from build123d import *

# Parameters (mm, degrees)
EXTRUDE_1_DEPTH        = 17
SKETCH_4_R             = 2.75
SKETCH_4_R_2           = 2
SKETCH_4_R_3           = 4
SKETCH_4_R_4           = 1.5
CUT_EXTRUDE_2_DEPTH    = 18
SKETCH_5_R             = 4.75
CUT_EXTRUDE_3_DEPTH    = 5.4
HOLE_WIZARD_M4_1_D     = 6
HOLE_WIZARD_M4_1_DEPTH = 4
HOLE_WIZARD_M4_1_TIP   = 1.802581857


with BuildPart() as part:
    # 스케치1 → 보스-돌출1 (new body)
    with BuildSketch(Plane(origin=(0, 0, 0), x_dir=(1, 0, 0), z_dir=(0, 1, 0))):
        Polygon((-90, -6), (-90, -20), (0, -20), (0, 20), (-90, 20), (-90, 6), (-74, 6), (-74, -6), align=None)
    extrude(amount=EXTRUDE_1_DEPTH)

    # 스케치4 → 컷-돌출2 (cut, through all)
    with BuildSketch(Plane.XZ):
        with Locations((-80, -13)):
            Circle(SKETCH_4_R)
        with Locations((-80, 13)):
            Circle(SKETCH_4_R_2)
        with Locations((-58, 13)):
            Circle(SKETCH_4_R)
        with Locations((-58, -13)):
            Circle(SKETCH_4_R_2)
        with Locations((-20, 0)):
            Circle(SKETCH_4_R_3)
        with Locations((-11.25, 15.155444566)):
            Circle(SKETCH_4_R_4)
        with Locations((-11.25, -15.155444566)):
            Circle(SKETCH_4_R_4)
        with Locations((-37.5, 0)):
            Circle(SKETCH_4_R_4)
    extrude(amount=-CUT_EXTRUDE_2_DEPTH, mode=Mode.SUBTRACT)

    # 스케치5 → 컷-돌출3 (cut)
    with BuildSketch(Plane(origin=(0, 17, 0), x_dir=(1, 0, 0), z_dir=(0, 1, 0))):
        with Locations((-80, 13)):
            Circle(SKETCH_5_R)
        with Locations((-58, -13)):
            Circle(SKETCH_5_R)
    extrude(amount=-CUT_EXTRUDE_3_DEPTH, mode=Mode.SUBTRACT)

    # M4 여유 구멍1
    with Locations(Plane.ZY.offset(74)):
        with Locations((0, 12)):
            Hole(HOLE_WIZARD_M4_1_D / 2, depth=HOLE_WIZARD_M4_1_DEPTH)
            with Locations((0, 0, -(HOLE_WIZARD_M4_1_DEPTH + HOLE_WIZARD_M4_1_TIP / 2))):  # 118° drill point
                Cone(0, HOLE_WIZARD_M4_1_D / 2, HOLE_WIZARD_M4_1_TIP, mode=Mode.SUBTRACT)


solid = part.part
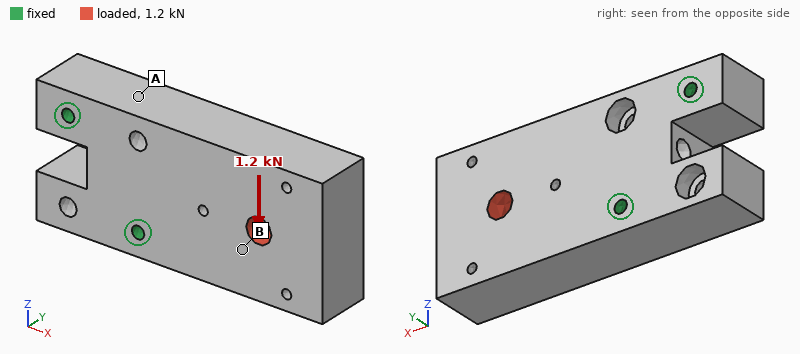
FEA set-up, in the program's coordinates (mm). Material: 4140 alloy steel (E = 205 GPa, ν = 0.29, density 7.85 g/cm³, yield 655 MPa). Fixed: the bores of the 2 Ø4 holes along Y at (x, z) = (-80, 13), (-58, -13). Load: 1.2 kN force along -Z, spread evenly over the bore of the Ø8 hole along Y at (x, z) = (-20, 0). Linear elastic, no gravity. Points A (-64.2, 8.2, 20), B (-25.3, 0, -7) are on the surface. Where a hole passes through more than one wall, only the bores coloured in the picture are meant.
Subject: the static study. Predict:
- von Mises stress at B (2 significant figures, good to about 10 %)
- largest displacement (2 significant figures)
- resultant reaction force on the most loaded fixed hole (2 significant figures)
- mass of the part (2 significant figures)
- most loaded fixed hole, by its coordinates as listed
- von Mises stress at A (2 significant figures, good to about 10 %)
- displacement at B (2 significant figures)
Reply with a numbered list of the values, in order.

1. 3.6 MPa
2. 6.0 µm
3. 2.0 kN
4. 430 g
5. (-58, -13)
6. 13 MPa
7. 3.2 µm
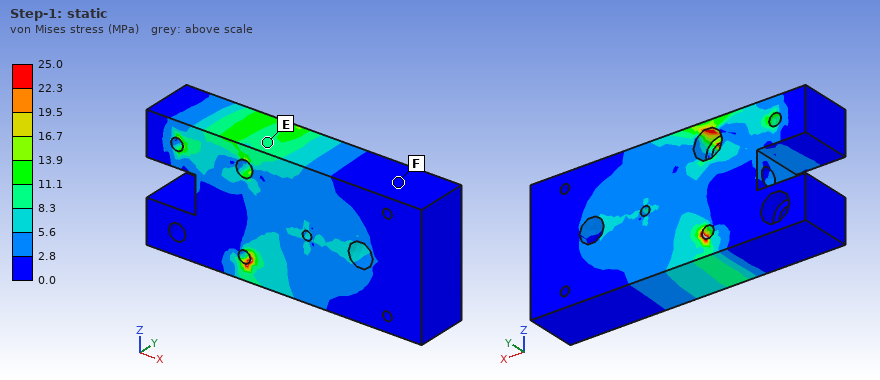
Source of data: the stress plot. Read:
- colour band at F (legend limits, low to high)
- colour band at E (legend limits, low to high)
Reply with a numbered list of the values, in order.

1. 0.0 to 2.8 MPa
2. 8.3 to 11.1 MPa
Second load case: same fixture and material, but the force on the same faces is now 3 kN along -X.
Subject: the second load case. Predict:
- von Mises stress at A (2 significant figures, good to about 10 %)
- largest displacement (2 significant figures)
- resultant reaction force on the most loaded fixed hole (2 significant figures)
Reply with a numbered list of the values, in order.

1. 10.0 MPa
2. 2.4 µm
3. 1.6 kN
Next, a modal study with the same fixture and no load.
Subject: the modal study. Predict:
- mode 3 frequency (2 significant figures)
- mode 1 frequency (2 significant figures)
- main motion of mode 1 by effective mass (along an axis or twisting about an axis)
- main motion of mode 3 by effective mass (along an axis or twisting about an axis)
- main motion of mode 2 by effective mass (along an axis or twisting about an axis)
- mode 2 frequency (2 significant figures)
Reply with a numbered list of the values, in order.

1. 8000 Hz
2. 3000 Hz
3. along Y
4. twisting about X
5. along Z
6. 5700 Hz
